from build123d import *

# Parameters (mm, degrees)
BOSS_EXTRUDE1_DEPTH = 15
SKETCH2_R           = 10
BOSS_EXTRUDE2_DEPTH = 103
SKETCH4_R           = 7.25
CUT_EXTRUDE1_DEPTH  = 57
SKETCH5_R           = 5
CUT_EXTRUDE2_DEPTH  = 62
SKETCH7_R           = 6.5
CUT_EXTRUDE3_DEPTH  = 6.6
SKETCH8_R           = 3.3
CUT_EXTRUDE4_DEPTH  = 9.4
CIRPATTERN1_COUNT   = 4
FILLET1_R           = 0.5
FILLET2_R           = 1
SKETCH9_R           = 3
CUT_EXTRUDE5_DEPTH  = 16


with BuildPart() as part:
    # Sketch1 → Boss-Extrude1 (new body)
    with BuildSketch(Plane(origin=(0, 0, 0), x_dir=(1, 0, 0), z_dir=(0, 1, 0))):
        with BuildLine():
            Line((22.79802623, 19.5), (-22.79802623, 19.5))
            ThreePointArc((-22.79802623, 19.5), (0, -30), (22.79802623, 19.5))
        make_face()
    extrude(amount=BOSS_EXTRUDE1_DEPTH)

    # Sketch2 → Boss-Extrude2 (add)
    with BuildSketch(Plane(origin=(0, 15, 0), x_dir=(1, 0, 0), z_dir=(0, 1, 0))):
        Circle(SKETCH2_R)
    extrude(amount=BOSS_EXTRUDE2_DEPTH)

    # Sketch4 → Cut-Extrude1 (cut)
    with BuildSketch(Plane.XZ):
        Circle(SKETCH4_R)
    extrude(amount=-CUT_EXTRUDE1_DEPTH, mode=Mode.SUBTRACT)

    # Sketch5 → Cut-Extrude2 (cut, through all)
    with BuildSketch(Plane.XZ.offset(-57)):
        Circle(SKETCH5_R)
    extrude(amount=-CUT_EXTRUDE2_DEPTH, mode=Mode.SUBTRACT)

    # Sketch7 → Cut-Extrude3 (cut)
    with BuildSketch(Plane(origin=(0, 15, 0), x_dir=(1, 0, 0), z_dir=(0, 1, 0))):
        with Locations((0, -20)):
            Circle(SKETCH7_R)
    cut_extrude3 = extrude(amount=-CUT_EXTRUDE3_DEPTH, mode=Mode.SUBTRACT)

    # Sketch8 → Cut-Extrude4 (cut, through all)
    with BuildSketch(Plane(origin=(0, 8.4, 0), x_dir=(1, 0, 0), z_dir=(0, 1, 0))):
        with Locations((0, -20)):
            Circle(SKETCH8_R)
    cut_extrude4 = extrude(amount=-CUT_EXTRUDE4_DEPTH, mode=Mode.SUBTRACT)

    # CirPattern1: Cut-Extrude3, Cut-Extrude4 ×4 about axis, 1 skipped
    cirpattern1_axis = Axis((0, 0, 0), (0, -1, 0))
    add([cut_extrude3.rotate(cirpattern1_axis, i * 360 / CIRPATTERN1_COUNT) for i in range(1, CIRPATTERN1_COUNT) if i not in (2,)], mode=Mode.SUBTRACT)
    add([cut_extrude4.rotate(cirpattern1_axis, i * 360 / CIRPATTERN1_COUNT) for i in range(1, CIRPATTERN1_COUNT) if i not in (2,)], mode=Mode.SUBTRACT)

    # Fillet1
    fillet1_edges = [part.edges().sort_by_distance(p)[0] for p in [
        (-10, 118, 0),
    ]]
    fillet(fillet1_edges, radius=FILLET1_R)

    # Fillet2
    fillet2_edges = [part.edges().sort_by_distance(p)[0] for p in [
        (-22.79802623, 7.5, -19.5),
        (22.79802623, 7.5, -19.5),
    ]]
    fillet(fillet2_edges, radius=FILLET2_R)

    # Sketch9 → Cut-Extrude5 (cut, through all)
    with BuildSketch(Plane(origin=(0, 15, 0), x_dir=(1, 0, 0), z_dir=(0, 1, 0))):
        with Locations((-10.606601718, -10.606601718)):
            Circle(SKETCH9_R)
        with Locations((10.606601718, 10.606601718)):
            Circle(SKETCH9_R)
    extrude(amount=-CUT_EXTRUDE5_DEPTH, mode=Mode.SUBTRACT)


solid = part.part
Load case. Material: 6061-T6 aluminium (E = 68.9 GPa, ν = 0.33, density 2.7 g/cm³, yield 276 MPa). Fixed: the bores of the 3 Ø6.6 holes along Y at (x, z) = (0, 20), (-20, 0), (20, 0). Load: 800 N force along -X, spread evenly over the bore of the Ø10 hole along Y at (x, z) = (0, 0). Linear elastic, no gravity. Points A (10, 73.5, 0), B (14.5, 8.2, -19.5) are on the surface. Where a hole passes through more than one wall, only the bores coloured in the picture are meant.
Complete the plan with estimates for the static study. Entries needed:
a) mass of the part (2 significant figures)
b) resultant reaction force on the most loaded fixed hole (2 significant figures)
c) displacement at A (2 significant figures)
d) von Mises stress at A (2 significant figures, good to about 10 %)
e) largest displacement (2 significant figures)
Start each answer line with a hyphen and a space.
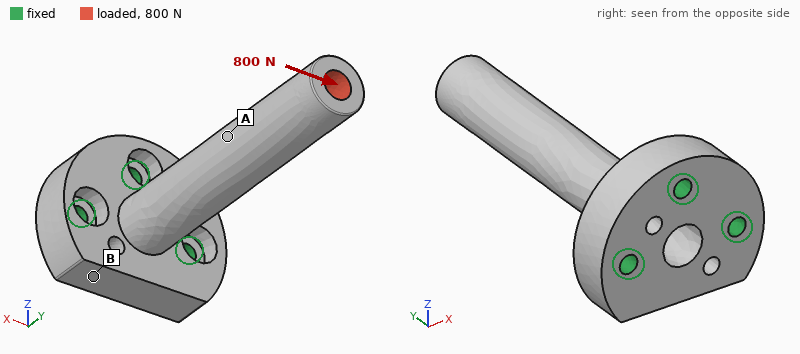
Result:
- 140 g
- 1.9 kN
- 0.26 mm
- 17 MPa
- 0.53 mm
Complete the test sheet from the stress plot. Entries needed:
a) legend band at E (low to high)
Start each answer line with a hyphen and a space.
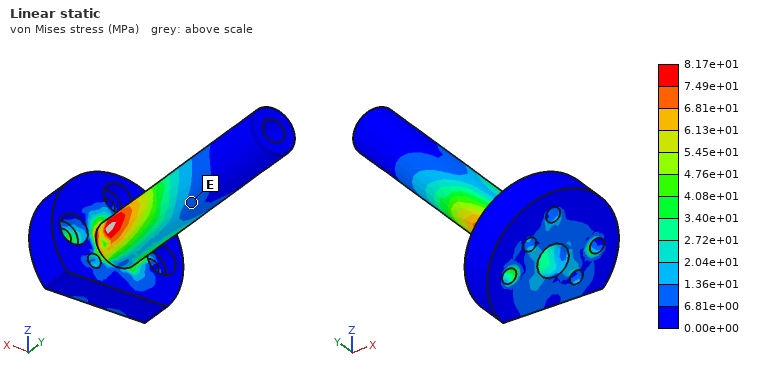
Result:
- 6.81e+00 to 1.36e+01 MPa
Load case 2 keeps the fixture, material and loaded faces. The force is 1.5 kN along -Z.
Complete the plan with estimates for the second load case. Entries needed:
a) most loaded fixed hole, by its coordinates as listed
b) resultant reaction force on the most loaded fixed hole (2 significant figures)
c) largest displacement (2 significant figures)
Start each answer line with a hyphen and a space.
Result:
- (0, 20)
- 4.6 kN
- 1.1 mm
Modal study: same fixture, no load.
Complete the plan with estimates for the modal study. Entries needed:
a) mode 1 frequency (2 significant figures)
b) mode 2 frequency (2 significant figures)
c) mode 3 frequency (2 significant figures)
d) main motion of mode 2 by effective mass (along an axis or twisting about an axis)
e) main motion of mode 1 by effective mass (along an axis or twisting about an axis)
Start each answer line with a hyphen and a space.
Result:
- 1100 Hz
- 1200 Hz
- 6500 Hz
- along X
- along Z
